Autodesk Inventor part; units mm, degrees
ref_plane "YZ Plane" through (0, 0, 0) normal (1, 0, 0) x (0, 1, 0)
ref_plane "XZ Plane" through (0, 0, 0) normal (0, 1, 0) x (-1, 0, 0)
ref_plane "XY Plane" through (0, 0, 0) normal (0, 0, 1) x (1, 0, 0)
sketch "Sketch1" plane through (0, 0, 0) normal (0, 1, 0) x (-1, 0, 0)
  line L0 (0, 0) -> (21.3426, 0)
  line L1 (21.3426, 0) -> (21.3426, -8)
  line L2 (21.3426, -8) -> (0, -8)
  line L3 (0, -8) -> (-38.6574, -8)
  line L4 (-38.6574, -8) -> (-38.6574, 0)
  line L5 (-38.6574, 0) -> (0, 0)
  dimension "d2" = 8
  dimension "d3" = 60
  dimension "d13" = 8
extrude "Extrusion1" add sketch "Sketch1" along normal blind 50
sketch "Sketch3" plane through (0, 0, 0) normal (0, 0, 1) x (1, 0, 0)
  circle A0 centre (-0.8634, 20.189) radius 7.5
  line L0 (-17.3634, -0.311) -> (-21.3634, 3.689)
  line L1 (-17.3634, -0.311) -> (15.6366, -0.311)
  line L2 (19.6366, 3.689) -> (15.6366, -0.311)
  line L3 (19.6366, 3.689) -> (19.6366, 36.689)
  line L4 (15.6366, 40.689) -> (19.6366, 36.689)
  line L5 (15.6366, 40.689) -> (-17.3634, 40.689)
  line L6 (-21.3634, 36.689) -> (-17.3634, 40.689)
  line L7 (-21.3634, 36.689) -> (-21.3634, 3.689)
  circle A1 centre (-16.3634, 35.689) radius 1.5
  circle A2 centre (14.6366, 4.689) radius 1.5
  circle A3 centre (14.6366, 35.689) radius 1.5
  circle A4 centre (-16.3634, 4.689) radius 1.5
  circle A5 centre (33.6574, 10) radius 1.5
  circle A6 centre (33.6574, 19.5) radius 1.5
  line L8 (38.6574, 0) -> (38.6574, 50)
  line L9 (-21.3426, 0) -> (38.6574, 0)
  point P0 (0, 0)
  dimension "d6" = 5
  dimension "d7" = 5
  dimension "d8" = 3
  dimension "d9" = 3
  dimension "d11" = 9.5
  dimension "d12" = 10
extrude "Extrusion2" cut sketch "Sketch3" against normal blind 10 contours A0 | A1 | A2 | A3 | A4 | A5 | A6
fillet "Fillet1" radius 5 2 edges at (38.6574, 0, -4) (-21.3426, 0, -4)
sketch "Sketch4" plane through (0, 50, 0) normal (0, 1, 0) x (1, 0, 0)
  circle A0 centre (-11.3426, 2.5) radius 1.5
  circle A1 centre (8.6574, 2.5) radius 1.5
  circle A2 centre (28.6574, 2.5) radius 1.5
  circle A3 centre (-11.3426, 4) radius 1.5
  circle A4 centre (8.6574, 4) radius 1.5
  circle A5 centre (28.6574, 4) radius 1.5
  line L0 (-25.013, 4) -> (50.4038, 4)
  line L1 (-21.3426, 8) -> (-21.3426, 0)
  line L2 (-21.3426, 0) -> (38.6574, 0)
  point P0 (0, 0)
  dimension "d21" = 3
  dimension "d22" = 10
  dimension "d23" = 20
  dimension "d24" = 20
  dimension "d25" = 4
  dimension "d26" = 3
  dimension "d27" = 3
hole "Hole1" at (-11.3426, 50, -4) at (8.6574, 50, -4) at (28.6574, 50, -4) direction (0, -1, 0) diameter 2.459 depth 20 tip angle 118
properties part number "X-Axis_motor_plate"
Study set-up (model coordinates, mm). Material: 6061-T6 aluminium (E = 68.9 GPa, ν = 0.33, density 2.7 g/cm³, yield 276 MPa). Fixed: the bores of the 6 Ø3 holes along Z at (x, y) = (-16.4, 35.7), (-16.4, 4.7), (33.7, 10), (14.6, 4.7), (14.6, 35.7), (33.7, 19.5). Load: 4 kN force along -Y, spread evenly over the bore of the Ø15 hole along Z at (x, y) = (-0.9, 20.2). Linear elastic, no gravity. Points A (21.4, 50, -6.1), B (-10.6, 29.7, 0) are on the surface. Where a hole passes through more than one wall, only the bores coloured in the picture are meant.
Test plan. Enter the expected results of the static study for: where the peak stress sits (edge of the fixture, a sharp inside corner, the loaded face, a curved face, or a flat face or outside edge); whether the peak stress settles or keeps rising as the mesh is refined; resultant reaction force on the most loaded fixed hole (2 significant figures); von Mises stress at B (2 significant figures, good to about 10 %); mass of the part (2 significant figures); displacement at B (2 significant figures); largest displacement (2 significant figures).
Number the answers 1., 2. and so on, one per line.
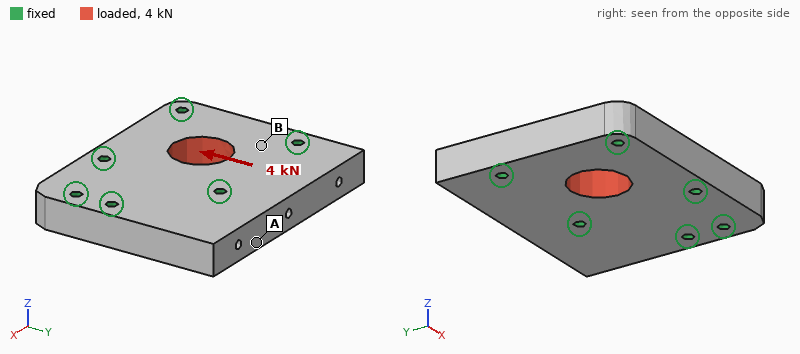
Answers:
1. edge of the fixture
2. keeps rising
3. 1.1 kN
4. 12 MPa
5. 59 g
6. 1.7 µm
7. 4.5 µm
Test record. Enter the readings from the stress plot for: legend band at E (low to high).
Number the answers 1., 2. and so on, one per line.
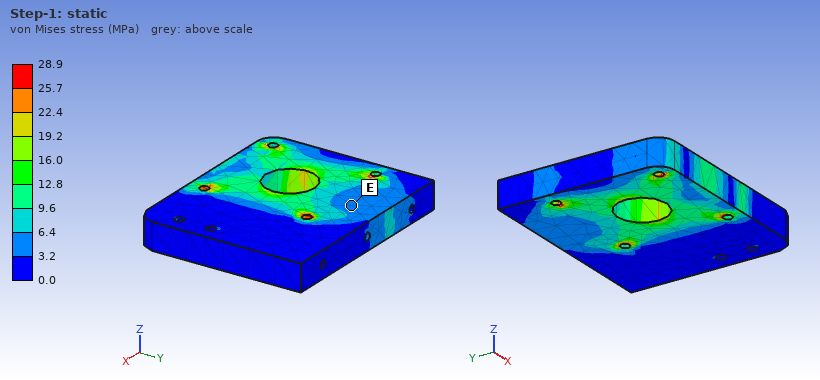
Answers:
1. 3.2 to 6.4 MPa
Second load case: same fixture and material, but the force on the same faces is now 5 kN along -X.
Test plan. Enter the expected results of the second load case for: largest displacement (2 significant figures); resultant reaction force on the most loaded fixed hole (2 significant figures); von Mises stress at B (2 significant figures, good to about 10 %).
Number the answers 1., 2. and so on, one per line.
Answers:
1. 5.7 µm
2. 1.2 kN
3. 16 MPa
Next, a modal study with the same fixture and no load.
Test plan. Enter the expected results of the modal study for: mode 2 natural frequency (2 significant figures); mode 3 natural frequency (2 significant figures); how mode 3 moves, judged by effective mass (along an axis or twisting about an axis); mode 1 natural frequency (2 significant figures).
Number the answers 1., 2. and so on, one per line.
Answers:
1. 19 kHz
2. 25 kHz
3. along Z
4. 13 kHz
